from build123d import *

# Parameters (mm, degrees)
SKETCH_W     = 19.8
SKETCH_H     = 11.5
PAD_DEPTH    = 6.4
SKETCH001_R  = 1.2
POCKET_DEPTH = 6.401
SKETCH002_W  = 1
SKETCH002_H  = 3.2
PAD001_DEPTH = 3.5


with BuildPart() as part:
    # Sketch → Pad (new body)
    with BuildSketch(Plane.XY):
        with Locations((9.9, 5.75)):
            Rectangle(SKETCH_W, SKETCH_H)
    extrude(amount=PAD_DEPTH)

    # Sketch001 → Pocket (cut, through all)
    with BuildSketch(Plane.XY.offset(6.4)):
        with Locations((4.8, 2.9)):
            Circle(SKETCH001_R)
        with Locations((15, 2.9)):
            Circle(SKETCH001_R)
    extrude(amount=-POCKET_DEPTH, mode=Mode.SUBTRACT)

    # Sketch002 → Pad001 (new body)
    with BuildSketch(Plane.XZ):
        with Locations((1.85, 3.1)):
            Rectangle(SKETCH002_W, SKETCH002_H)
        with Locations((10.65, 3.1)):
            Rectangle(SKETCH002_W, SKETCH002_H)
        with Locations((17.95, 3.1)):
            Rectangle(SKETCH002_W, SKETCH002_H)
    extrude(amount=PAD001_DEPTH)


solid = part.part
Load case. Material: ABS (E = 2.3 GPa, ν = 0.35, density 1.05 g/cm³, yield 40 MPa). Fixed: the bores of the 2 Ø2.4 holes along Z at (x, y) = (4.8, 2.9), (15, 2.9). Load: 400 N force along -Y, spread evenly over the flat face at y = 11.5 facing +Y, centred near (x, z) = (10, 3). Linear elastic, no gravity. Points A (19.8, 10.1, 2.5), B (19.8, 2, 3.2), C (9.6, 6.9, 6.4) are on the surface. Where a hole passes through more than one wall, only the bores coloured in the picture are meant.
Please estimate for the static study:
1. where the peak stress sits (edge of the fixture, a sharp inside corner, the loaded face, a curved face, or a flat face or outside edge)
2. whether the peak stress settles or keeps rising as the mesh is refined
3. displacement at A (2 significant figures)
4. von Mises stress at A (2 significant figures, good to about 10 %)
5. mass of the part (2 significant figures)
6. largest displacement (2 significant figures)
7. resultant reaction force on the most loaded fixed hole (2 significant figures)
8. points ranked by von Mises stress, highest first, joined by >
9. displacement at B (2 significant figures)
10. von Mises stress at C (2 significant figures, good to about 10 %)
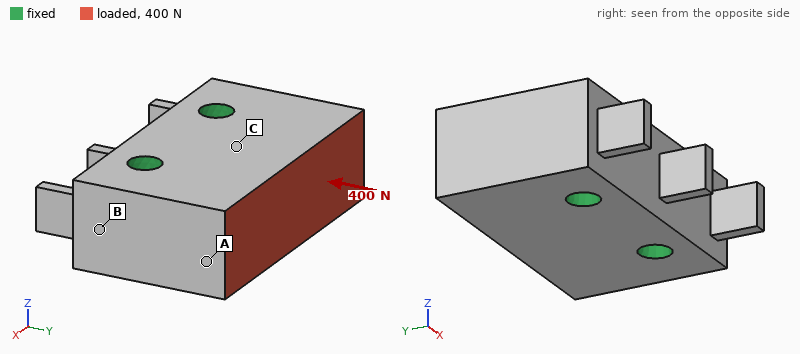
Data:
edge of the fixture
keeps rising
15 µm
3.1 MPa
1.5 g
18 µm
200 N
A > C > B
8.3 µm
2.0 MPa
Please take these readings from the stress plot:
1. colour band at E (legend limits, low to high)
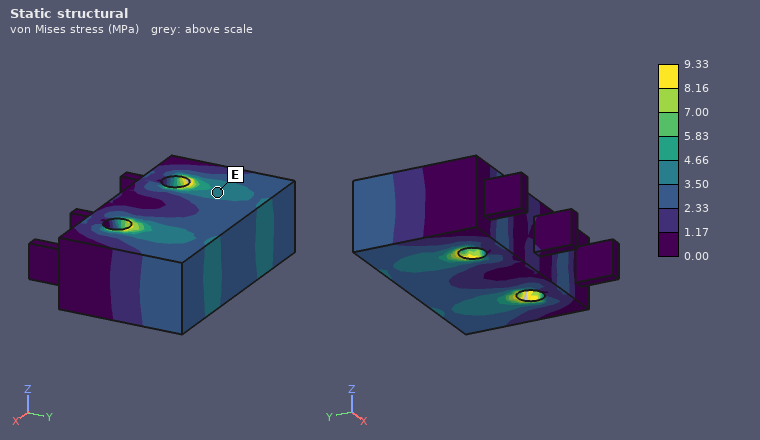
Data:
3.50 to 4.66 MPa
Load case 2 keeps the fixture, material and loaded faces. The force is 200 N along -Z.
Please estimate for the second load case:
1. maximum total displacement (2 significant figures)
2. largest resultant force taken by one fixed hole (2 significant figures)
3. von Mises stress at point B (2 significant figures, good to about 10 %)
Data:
77 µm
100 N
3.2 MPa
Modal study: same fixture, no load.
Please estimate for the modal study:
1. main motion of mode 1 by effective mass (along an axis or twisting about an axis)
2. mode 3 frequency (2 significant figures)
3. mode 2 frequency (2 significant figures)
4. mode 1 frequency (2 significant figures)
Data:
along Z
17 kHz
16 kHz
14 kHz
